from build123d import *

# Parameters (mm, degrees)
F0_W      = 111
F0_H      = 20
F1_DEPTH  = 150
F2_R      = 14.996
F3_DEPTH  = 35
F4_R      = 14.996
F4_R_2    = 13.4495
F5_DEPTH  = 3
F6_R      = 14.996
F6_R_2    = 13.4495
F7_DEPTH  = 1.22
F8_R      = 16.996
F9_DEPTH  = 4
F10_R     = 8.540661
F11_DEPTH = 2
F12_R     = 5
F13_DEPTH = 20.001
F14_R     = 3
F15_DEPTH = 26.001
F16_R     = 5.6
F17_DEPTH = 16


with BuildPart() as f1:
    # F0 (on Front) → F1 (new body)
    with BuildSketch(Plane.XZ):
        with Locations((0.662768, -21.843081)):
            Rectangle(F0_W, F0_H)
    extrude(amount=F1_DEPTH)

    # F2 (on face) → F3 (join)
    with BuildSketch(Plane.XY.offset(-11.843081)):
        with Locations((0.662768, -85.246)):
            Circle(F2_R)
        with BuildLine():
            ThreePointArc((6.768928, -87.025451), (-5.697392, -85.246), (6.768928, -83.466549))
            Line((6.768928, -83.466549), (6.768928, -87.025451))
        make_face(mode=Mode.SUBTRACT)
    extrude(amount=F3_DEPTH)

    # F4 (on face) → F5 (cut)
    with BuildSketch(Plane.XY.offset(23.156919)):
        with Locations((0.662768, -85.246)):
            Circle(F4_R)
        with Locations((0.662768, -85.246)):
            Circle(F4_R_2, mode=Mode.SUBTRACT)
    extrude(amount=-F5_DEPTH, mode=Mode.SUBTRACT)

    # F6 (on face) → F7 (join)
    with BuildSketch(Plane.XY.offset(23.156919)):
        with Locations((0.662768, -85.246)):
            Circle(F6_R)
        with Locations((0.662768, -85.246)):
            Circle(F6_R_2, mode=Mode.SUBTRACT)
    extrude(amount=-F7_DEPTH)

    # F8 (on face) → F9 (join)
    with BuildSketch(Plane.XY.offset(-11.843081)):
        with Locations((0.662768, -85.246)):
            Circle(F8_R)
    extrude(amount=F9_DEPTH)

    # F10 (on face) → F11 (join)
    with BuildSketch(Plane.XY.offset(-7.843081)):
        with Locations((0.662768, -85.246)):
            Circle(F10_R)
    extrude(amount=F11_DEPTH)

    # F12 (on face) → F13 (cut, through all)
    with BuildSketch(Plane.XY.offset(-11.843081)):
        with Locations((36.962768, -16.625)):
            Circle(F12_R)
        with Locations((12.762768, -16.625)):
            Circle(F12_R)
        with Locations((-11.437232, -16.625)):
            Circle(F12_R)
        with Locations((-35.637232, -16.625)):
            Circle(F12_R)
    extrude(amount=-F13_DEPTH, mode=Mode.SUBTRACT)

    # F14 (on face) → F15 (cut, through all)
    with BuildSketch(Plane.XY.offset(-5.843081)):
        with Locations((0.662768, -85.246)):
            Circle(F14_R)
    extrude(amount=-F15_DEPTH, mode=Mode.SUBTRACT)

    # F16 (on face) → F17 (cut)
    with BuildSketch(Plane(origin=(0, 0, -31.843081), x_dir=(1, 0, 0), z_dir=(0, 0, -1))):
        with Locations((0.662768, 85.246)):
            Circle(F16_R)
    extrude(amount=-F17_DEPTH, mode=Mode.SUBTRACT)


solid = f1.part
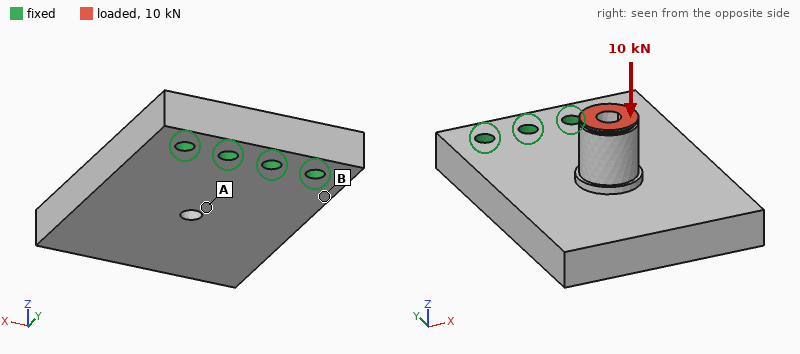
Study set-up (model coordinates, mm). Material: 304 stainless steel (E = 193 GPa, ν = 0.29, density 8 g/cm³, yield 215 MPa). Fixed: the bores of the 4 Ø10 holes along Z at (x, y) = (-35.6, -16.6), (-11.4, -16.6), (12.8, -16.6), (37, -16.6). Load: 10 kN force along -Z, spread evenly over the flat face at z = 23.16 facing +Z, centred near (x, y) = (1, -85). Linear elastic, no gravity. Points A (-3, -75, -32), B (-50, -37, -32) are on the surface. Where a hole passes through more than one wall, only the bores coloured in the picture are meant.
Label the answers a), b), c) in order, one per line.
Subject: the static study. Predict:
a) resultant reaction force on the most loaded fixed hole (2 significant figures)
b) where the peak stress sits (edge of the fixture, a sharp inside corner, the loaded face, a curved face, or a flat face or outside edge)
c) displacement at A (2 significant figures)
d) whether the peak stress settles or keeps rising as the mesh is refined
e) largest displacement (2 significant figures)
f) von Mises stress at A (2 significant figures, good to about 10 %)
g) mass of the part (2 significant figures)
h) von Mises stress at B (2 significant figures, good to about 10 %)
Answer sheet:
a) 3.3 kN
b) edge of the fixture
c) 0.061 mm
d) keeps rising
e) 0.18 mm
f) 16 MPa
g) 2.8 kg
h) 56 MPa
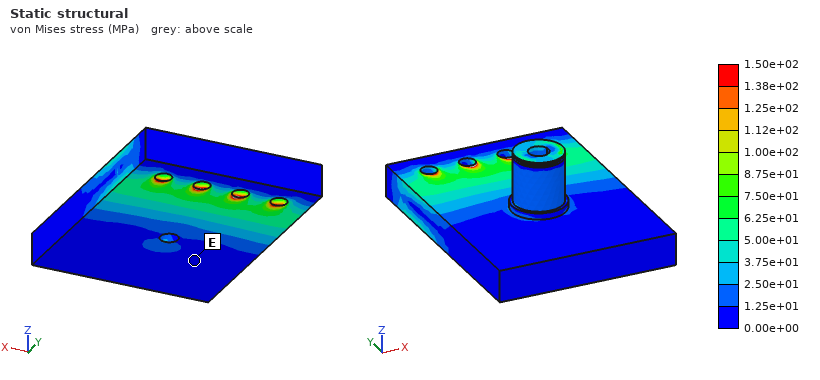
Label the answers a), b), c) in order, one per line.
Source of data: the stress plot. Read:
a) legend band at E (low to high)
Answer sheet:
a) 0.00e+00 to 1.25e+01 MPa
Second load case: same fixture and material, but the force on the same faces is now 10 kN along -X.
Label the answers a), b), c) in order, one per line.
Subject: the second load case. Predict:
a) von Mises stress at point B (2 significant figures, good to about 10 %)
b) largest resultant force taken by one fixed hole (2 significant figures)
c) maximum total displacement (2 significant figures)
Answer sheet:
a) 33 MPa
b) 9.6 kN
c) 94 µm
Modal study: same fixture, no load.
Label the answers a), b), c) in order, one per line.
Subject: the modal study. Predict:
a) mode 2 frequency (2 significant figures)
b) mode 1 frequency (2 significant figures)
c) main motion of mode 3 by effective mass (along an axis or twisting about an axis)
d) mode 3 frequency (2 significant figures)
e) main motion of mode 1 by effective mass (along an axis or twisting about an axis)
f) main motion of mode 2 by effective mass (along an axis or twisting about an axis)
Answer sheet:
a) 2300 Hz
b) 890 Hz
c) along X
d) 3200 Hz
e) along Z
f) twisting about Y
